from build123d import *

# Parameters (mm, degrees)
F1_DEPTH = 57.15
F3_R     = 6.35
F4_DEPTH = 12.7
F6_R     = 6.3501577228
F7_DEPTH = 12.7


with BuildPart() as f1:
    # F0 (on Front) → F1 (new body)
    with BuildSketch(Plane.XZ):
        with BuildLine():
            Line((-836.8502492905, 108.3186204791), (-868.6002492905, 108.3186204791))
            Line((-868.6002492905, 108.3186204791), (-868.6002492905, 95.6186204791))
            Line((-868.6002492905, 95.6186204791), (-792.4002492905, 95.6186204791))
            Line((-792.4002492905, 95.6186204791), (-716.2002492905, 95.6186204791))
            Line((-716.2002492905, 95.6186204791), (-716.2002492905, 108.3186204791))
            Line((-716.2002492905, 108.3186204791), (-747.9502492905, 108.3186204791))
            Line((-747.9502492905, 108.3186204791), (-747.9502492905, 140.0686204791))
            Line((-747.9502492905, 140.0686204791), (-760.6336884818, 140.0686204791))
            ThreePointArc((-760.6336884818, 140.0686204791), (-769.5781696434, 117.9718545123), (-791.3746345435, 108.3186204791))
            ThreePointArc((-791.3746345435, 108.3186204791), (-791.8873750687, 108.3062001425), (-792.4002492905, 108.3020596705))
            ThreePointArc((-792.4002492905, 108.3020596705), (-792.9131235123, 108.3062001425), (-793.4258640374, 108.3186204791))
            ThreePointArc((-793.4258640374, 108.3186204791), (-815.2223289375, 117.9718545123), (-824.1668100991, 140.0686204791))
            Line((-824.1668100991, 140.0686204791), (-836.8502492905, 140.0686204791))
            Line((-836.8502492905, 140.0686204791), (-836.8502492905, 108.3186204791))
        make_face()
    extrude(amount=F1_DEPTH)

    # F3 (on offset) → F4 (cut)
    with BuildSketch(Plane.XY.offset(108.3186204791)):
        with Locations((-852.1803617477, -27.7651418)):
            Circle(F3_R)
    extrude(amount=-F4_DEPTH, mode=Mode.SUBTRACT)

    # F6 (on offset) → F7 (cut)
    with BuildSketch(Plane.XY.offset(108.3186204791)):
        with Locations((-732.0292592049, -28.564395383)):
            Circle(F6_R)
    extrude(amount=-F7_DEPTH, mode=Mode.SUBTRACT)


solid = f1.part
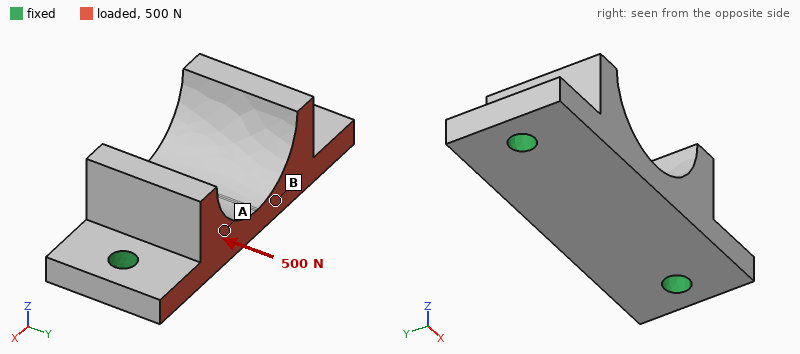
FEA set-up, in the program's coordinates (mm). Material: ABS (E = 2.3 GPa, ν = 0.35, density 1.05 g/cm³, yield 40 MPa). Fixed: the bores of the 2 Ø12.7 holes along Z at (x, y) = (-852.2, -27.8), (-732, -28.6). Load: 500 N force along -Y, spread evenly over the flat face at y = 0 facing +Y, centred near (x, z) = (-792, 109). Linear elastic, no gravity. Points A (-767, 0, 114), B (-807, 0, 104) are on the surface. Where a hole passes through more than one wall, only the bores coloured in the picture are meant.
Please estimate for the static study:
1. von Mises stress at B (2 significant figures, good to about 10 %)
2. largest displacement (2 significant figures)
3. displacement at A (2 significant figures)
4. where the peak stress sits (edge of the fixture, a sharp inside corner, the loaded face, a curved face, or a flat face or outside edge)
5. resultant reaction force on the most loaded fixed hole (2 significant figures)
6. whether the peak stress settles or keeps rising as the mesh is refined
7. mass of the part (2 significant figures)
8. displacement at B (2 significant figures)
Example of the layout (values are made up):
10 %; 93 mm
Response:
0.47 MPa; 59 µm; 40 µm; edge of the fixture; 250 N; keeps rising; 190 g; 33 µm
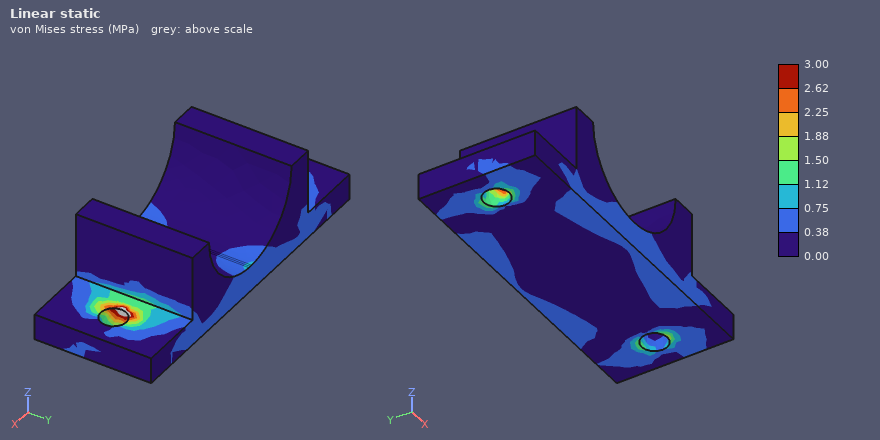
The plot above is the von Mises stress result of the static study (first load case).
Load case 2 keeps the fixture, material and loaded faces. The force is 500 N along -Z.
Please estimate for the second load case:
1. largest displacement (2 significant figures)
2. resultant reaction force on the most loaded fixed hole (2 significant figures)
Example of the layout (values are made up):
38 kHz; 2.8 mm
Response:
0.20 mm; 260 N
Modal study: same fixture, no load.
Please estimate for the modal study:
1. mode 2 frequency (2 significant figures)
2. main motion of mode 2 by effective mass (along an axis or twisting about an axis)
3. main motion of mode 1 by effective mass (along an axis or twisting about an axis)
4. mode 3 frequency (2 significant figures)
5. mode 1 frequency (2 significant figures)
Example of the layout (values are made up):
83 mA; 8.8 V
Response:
1100 Hz; along Y; along Z; 1800 Hz; 990 Hz
